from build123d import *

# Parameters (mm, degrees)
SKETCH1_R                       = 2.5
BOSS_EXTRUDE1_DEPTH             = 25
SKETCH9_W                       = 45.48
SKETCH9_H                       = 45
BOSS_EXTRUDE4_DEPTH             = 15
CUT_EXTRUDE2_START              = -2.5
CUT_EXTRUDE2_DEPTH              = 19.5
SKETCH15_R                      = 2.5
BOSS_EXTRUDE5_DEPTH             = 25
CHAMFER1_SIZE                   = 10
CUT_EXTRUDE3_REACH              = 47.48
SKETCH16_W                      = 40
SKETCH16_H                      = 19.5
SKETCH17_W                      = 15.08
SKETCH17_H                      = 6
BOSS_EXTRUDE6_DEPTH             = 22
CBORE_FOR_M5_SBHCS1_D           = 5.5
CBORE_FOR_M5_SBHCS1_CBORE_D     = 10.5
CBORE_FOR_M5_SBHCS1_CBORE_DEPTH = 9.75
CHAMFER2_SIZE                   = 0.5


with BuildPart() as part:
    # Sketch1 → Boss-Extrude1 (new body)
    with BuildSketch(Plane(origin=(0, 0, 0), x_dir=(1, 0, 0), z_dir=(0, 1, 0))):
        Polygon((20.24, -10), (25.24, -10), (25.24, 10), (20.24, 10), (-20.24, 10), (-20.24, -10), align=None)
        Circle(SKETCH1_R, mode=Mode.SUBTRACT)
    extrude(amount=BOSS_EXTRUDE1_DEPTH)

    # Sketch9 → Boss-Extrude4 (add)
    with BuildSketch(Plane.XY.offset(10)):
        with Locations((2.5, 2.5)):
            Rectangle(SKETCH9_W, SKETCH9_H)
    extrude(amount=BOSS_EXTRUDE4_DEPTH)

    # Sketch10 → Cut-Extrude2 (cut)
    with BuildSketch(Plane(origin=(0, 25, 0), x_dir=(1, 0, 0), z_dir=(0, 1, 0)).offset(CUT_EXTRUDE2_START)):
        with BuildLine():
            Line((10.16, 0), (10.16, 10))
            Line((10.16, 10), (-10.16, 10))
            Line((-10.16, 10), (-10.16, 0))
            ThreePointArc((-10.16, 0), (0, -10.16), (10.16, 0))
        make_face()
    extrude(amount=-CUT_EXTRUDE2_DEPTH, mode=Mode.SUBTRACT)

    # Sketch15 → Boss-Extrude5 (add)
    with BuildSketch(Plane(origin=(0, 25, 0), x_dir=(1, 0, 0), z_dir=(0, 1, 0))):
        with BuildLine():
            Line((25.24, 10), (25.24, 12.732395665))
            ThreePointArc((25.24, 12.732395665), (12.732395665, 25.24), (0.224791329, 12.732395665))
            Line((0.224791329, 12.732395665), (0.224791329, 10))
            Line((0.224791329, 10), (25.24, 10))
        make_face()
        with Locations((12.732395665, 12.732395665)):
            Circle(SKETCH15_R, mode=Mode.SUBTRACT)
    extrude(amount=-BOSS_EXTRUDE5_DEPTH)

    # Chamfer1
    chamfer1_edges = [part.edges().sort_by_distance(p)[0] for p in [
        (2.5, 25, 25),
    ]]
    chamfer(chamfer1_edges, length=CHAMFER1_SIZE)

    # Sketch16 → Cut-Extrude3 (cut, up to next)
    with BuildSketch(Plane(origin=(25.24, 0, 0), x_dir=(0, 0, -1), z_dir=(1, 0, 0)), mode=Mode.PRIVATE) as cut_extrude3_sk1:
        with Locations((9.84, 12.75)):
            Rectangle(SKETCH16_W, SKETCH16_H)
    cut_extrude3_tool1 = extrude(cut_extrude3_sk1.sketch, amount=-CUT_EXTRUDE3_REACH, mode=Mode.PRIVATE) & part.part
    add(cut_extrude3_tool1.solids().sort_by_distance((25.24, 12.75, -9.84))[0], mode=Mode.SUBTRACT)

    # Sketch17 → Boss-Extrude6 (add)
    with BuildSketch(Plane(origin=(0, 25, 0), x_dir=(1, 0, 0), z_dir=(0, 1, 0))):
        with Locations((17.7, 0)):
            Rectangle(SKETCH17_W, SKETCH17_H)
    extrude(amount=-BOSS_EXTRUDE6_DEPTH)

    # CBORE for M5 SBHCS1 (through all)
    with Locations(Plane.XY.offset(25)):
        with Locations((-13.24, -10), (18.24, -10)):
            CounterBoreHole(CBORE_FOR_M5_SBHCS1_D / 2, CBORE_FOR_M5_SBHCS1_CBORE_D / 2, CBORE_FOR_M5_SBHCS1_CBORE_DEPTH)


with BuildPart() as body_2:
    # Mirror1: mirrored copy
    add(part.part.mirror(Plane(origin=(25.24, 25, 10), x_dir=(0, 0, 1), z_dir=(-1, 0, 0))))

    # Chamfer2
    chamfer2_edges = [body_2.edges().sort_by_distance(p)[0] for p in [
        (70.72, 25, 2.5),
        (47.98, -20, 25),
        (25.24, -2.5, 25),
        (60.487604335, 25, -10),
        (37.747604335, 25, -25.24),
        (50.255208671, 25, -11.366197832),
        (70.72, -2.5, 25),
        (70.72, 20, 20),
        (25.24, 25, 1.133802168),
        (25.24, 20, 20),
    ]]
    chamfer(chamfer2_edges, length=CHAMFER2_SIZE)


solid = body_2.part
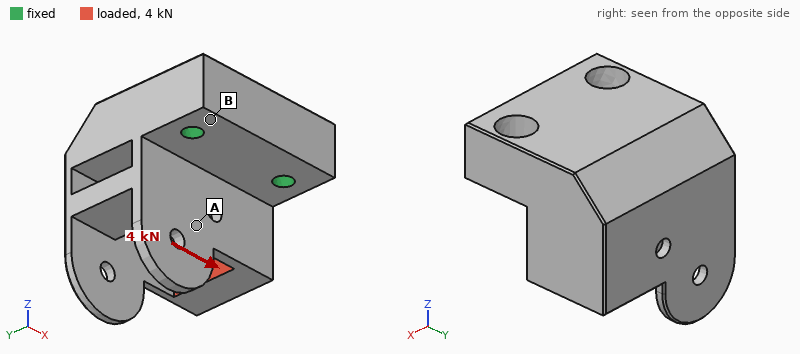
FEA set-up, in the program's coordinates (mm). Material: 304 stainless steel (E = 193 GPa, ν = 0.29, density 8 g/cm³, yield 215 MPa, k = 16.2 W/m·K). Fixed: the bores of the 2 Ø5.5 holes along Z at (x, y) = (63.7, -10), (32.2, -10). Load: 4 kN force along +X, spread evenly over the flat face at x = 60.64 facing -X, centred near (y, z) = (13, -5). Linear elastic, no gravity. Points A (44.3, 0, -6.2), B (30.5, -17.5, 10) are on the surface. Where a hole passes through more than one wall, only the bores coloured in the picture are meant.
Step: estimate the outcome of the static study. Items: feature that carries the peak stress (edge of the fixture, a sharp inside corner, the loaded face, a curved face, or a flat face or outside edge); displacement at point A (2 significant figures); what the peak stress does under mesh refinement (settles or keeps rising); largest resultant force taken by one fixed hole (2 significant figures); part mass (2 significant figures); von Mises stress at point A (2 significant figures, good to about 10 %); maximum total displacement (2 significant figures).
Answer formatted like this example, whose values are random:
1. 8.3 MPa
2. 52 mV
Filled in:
1. edge of the fixture
2. 14 µm
3. keeps rising
4. 3.9 kN
5. 310 g
6. 34 MPa
7. 36 µm
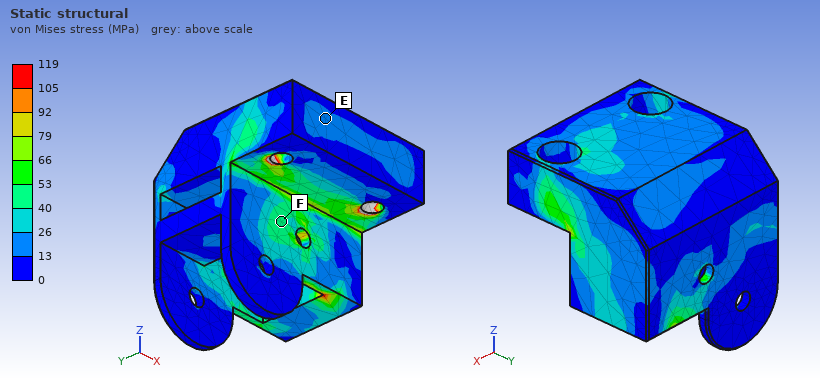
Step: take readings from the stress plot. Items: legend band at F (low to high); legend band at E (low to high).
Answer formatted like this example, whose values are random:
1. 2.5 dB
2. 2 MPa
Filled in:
1. 40 to 53 MPa
2. 13 to 26 MPa
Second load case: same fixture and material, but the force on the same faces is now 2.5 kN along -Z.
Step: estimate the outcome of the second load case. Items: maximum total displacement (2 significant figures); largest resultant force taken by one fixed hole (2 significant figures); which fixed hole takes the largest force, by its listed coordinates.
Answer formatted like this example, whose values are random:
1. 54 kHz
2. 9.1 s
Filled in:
1. 68 µm
2. 2.2 kN
3. (63.7, -10)
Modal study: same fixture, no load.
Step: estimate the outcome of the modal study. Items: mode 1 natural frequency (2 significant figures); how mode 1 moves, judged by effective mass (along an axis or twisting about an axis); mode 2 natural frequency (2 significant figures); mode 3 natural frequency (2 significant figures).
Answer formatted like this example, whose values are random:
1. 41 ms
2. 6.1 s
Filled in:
1. 2600 Hz
2. along Z
3. 4300 Hz
4. 4900 Hz
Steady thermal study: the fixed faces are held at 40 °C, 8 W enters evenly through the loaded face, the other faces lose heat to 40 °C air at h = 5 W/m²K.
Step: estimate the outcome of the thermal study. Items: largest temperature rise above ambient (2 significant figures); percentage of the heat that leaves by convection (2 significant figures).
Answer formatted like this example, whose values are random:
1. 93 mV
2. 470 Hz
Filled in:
1. 56 K
2. 14 %
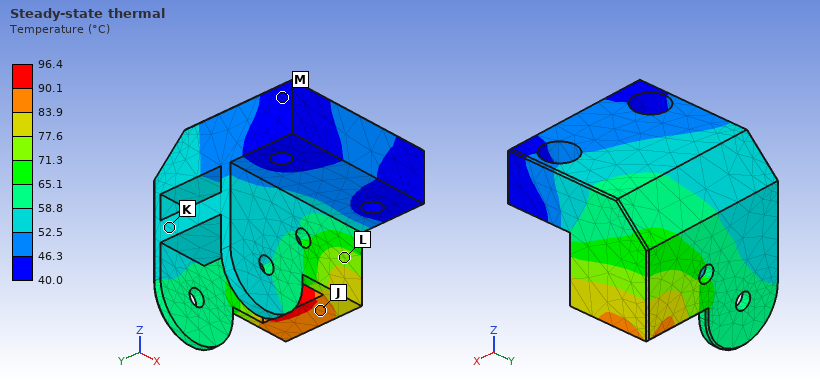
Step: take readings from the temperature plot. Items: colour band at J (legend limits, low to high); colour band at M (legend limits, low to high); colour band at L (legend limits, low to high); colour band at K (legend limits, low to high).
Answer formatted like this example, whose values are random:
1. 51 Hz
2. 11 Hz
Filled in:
1. 83.9 to 90.1 °C
2. 40.0 to 46.3 °C
3. 71.3 to 77.6 °C
4. 52.5 to 58.8 °C
